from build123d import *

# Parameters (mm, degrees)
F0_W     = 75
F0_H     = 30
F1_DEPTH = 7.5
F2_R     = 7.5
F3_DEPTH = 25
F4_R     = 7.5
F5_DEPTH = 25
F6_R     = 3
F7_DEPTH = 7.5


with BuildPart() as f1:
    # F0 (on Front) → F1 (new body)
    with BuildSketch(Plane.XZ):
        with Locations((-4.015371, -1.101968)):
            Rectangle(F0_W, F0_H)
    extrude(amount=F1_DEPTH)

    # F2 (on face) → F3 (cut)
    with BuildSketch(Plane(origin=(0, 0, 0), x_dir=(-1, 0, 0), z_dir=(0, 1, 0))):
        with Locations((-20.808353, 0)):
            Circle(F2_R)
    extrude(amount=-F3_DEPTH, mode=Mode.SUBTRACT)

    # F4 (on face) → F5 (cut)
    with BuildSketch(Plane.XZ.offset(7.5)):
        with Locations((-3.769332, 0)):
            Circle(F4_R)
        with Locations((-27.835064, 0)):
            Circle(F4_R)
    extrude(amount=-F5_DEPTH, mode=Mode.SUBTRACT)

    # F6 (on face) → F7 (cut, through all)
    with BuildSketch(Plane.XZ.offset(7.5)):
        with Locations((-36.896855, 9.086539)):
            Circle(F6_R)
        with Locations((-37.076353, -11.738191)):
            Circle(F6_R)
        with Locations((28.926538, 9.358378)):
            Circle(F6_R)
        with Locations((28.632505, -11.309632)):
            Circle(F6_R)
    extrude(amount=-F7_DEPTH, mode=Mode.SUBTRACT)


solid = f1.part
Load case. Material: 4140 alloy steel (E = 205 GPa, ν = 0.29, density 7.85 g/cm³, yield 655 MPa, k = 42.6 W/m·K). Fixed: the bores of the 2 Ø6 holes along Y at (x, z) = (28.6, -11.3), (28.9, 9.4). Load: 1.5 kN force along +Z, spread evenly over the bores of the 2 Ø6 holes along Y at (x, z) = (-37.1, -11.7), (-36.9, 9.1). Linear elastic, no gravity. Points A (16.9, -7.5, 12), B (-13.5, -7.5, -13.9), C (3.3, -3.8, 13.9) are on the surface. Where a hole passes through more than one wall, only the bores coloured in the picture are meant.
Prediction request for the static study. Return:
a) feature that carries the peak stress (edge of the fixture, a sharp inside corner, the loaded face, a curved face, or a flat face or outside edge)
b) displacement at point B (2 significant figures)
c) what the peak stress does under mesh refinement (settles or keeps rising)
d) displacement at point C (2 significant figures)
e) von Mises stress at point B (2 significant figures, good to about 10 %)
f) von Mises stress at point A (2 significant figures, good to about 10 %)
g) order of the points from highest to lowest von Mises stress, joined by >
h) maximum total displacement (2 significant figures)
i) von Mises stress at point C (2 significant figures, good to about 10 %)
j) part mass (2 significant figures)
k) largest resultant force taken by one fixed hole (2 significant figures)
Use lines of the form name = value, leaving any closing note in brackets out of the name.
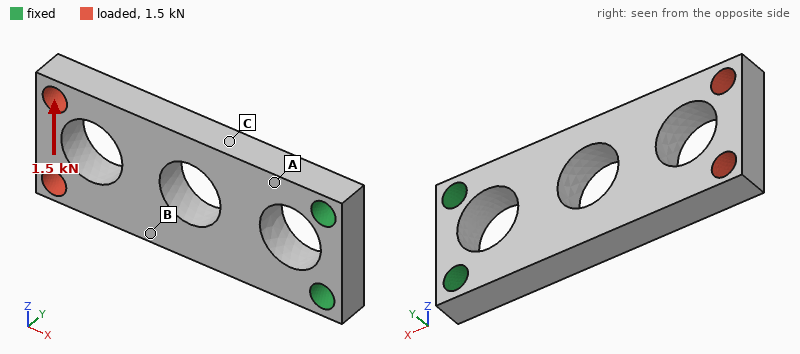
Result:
feature that carries the peak stress = edge of the fixture
displacement at point B = 36 µm
what the peak stress does under mesh refinement = keeps rising
displacement at point C = 18 µm
von Mises stress at point B = 25 MPa
von Mises stress at point A = 64 MPa
order of the points from highest to lowest von Mises stress, joined by > = C > A > B
maximum total displacement = 73 µm
von Mises stress at point C = 96 MPa
part mass = 95 g
largest resultant force taken by one fixed hole = 3.9 kN
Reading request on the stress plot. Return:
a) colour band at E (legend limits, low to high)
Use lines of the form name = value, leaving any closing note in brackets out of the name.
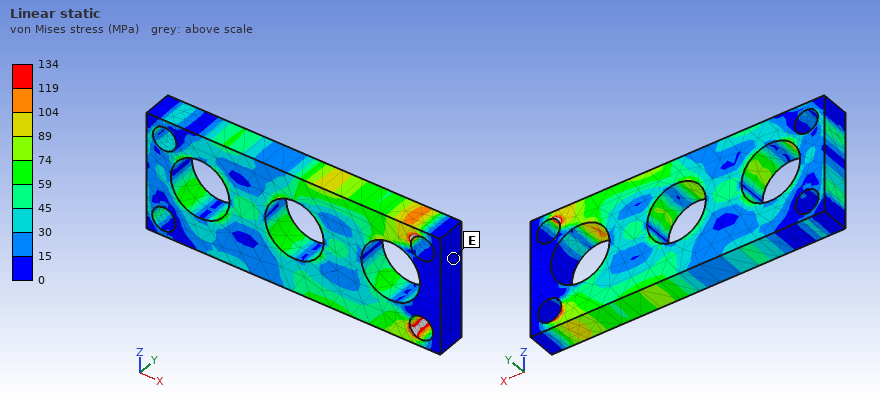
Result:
colour band at E = 0 to 15 MPa
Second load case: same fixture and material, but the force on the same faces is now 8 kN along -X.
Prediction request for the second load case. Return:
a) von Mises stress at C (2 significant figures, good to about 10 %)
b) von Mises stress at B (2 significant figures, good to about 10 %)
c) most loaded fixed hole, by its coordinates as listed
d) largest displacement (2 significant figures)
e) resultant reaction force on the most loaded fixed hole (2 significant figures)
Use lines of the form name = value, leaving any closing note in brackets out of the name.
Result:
von Mises stress at C = 70 MPa
von Mises stress at B = 66 MPa
most loaded fixed hole, by its coordinates as listed = (28.6, -11.3)
largest displacement = 28 µm
resultant reaction force on the most loaded fixed hole = 4.3 kN
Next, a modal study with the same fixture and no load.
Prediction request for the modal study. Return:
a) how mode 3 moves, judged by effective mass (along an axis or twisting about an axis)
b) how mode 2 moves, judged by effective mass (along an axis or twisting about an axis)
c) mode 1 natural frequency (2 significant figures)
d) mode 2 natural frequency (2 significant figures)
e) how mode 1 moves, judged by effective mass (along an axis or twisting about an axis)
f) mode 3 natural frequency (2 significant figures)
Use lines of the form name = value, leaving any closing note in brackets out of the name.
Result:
how mode 3 moves, judged by effective mass = twisting about X
how mode 2 moves, judged by effective mass = along Z
mode 1 natural frequency = 1200 Hz
mode 2 natural frequency = 4500 Hz
how mode 1 moves, judged by effective mass = along Y
mode 3 natural frequency = 4800 Hz
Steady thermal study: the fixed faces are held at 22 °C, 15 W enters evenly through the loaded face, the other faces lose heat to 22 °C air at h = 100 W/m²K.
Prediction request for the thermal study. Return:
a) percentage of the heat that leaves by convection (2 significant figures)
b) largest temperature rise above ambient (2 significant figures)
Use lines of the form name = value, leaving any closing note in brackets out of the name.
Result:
percentage of the heat that leaves by convection = 83 %
largest temperature rise above ambient = 64 K
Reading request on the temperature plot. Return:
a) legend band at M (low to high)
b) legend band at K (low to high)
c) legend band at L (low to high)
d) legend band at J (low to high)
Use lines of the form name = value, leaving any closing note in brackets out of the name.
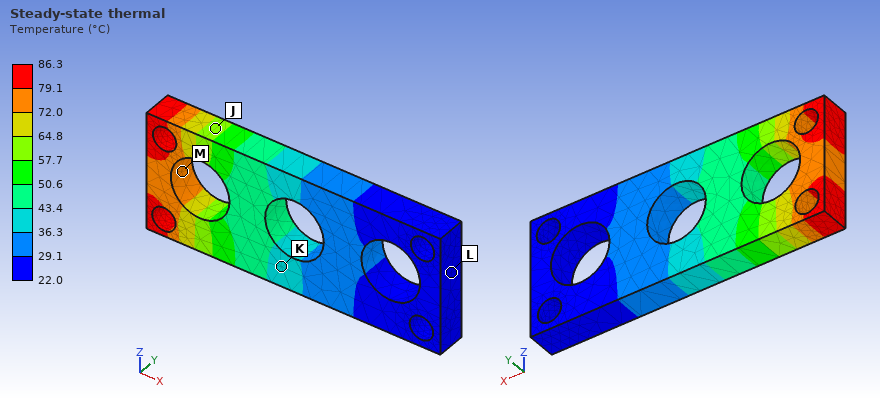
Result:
legend band at M = 72.0 to 79.1 °C
legend band at K = 36.3 to 43.4 °C
legend band at L = 22.0 to 29.1 °C
legend band at J = 57.7 to 64.8 °C
